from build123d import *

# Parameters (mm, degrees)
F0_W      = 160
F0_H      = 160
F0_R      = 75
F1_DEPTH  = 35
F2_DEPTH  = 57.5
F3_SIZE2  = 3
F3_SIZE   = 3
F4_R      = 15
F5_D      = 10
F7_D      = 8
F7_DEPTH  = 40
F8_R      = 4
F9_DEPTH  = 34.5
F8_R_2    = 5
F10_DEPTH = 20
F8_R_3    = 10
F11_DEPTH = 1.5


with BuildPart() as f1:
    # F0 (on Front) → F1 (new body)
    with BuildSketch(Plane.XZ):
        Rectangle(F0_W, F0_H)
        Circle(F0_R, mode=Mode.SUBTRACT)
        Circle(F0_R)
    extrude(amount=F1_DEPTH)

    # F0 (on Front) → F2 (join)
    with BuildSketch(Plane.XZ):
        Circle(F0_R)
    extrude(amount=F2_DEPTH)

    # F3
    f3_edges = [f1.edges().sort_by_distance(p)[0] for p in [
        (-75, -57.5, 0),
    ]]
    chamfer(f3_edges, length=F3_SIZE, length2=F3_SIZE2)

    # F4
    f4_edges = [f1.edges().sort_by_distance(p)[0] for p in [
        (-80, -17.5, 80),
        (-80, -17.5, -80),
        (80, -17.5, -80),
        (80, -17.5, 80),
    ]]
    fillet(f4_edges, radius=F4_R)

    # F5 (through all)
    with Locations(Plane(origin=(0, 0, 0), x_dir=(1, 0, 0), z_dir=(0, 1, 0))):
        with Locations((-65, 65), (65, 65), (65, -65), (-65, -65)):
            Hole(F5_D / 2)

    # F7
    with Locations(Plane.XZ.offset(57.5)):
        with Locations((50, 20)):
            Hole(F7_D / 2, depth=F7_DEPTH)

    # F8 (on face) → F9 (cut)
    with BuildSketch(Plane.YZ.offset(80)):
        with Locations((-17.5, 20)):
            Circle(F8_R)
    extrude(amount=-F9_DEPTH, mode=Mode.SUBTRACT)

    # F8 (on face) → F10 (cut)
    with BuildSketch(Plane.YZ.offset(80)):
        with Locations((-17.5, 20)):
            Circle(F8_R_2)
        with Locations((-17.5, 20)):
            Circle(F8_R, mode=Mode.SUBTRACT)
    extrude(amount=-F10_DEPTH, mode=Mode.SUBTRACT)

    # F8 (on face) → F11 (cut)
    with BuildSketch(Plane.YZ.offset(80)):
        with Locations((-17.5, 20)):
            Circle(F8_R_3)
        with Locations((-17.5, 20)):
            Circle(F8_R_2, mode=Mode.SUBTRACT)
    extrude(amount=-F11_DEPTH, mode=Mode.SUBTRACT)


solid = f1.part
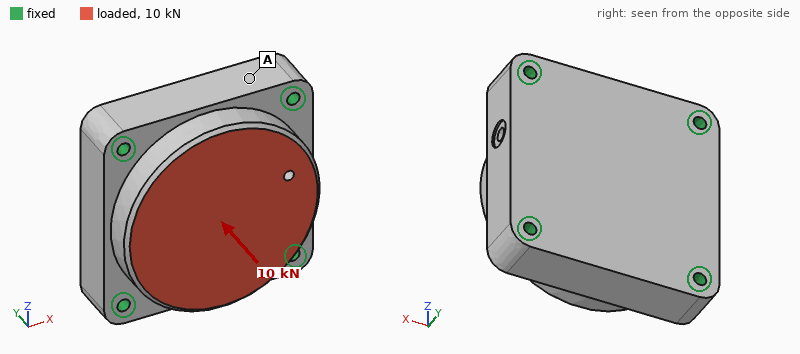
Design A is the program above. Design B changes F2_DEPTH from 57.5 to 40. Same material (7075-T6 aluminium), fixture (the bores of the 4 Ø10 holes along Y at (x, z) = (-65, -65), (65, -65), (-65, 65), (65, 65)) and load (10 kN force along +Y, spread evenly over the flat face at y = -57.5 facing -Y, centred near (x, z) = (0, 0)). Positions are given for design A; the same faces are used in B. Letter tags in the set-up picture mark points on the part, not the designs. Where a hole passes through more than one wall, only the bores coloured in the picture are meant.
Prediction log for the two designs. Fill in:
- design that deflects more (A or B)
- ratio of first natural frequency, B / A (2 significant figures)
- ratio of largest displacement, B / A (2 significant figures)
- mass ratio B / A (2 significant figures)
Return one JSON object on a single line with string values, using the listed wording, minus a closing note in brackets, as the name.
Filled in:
{"design that deflects more": "B", "ratio of first natural frequency, B / A": "1.00", "ratio of largest displacement, B / A": "1.6", "mass ratio B / A": "0.76"}
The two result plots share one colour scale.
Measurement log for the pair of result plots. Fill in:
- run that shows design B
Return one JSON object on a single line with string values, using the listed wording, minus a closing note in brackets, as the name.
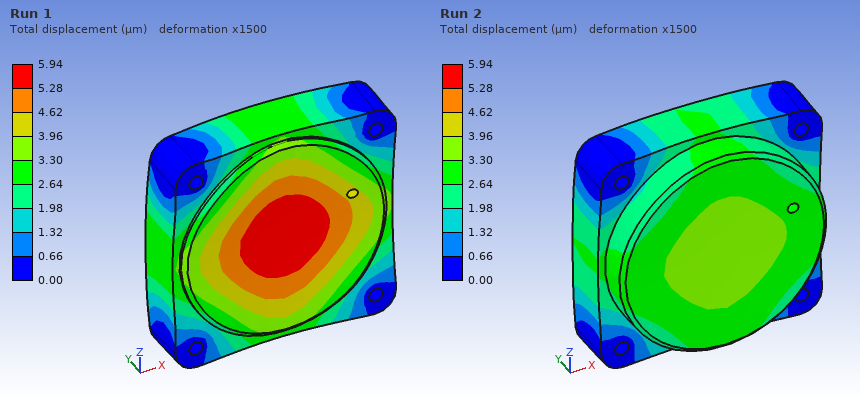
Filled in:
{"run that shows design B": "Run 1"}
